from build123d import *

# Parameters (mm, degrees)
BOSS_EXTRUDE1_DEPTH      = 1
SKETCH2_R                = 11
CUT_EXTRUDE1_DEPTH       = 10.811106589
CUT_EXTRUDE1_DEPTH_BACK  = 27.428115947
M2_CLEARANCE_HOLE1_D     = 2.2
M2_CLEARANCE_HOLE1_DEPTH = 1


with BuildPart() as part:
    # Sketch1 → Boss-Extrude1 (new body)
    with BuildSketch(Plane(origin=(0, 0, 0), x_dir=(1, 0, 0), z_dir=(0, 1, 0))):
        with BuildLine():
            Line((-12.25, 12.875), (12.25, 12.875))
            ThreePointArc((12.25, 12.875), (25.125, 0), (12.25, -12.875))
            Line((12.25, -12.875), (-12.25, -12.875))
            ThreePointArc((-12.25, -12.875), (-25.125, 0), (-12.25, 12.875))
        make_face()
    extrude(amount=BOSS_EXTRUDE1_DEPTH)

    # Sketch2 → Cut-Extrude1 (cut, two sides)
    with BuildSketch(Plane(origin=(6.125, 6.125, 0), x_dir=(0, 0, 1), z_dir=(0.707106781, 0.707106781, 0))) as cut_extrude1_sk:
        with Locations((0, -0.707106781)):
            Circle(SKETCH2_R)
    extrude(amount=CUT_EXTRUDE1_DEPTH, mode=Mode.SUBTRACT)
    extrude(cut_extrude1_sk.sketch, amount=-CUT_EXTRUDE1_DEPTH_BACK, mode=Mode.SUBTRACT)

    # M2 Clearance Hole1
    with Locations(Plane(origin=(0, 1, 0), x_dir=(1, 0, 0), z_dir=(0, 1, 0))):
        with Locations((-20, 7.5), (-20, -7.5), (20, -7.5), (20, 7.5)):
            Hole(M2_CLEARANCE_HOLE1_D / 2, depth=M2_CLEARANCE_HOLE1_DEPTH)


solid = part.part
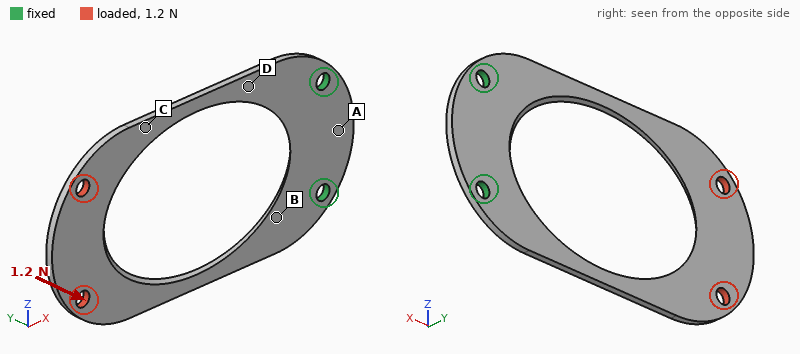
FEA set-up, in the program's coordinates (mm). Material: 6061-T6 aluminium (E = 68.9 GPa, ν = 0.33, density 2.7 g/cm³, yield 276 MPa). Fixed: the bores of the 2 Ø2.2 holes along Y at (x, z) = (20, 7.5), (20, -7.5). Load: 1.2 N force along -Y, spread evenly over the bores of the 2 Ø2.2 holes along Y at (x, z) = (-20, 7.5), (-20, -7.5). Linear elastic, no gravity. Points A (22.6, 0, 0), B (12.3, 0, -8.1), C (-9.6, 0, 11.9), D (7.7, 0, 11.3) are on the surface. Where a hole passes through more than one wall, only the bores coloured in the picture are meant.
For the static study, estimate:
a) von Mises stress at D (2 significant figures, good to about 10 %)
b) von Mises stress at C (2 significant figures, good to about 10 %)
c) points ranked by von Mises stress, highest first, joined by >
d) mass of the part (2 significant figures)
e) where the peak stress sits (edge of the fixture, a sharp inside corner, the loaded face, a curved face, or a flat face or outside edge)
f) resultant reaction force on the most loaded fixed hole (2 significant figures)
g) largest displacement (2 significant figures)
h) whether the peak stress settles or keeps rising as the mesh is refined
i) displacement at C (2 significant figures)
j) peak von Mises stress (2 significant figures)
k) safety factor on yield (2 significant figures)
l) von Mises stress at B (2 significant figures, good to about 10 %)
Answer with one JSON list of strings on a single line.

["29 MPa", "10 MPa", "D > B > C > A", "1.6 g", "a curved face", "0.70 N", "0.65 mm", "settles", "0.30 mm", "40 MPa", "6.9", "20 MPa"]
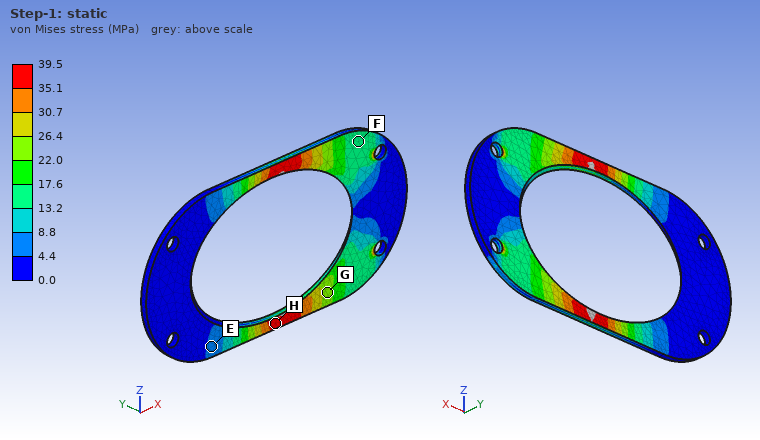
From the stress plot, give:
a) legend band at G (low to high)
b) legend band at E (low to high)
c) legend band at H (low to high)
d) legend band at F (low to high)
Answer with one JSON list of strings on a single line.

["22.0 to 26.4 MPa", "4.4 to 8.8 MPa", "35.1 to 39.5 MPa", "13.2 to 17.6 MPa"]
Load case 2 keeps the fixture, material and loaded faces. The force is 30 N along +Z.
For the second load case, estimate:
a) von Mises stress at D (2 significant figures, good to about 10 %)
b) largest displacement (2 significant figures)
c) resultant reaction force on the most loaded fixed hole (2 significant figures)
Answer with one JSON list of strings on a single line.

["13 MPa", "0.13 mm", "70 N"]
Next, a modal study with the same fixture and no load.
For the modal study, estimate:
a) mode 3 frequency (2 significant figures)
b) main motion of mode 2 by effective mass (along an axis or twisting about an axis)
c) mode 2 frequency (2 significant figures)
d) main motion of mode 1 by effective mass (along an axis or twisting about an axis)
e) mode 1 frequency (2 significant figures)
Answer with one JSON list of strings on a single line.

["2700 Hz", "twisting about X", "1200 Hz", "along Y", "320 Hz"]
